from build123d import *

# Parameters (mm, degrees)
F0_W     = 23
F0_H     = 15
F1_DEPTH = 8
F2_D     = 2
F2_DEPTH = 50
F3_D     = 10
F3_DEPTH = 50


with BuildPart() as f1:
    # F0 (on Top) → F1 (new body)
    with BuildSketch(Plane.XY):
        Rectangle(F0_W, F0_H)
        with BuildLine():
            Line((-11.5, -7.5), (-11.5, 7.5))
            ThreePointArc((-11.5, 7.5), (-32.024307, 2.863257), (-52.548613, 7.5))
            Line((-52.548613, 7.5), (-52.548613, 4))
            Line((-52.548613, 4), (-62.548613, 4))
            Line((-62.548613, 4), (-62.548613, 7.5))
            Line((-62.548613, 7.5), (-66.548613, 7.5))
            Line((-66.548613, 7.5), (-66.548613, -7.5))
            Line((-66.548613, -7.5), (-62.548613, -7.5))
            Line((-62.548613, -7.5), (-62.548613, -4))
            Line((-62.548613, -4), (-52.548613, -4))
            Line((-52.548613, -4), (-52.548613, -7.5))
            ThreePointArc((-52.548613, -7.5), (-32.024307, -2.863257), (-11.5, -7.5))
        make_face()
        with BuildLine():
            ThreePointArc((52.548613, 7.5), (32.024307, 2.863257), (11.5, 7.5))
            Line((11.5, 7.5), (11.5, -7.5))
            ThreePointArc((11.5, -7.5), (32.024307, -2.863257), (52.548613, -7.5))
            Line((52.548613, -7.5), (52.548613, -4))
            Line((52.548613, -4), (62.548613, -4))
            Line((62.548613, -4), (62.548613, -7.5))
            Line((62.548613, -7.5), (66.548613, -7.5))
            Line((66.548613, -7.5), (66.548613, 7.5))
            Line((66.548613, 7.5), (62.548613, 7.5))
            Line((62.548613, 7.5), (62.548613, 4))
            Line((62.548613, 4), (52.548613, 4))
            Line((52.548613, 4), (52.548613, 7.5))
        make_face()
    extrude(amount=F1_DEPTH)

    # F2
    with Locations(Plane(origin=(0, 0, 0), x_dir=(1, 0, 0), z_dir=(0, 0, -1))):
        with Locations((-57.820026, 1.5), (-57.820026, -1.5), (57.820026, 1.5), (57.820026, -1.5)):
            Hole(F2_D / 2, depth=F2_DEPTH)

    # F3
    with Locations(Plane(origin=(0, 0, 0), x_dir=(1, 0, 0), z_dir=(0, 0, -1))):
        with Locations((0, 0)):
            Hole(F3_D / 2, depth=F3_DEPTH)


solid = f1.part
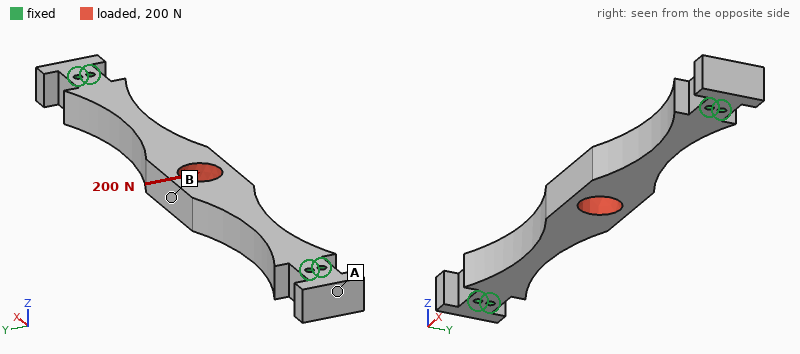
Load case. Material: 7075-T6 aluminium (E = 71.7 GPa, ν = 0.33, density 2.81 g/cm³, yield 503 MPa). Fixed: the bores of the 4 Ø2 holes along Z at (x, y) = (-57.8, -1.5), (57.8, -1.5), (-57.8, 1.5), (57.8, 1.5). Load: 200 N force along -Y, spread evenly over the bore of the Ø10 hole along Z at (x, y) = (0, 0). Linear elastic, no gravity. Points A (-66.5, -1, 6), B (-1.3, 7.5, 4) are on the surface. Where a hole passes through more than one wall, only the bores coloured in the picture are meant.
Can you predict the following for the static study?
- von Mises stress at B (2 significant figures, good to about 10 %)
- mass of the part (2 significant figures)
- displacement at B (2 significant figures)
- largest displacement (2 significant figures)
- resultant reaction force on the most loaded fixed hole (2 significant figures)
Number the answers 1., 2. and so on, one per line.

1. 13 MPa
2. 28 g
3. 35 µm
4. 35 µm
5. 530 N
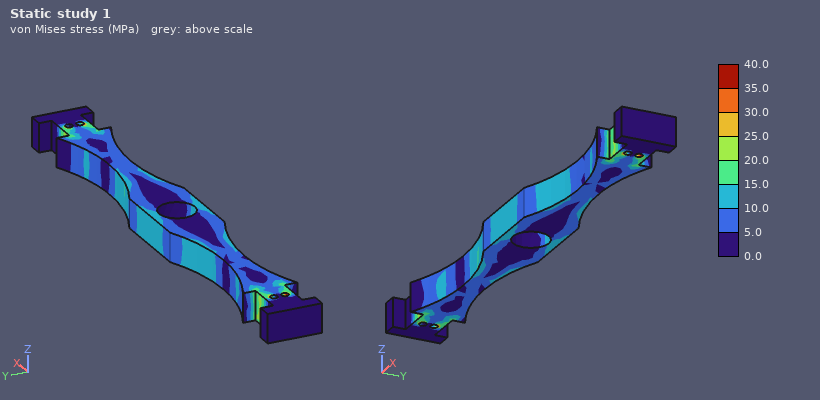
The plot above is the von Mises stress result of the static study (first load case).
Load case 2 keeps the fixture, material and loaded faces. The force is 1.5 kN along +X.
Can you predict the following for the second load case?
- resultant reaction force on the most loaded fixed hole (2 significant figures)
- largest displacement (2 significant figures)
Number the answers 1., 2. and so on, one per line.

1. 380 N
2. 8.9 µm
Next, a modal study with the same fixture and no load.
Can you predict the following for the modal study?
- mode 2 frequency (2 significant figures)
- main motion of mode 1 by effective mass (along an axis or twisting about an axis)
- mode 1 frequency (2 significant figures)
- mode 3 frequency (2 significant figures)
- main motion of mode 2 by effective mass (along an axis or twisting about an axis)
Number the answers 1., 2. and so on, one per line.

1. 3400 Hz
2. along Z
3. 2700 Hz
4. 7400 Hz
5. along Y
